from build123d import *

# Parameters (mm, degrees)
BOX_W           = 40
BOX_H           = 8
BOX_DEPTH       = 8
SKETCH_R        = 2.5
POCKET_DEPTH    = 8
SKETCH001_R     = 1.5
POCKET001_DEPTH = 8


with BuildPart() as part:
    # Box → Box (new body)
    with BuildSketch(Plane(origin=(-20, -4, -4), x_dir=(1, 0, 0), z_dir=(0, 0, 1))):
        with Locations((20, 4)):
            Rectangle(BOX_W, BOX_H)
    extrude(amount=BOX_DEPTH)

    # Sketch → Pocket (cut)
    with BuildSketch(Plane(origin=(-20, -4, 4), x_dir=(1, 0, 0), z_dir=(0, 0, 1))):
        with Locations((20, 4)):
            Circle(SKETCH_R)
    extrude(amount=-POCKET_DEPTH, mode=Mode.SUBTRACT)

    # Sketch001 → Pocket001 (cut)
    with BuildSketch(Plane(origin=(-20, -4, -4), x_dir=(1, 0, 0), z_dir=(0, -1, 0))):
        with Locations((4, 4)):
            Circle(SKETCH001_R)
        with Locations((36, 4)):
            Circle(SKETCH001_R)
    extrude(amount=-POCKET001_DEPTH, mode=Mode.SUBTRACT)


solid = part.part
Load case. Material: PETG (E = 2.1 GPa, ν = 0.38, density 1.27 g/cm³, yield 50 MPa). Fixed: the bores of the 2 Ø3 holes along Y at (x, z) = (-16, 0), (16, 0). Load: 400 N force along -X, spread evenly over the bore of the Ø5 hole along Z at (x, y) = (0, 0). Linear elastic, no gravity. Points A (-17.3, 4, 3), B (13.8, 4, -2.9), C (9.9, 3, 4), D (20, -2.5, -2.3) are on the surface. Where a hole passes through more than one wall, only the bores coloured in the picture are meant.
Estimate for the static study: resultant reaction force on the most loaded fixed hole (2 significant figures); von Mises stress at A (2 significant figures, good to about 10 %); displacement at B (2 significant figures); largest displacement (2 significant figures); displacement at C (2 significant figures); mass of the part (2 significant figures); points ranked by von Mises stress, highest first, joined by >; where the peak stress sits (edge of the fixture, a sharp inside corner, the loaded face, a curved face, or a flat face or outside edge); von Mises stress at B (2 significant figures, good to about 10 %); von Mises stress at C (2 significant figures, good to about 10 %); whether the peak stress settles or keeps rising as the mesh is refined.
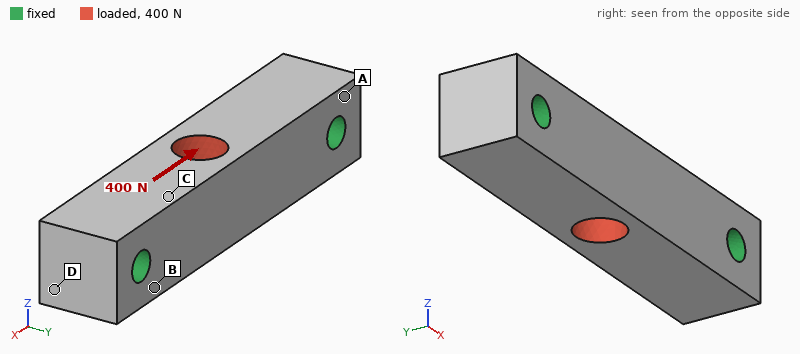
200 N
1.2 MPa
5.3 µm
24 µm
9.7 µm
2.9 g
C > B > A > D
edge of the fixture
2.0 MPa
2.8 MPa
keeps rising
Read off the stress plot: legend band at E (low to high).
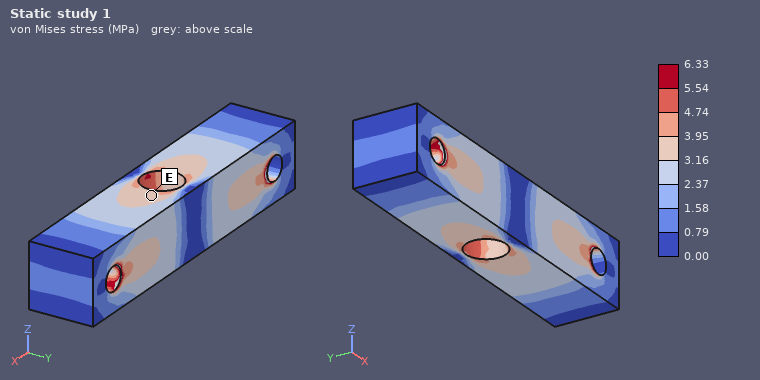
3.16 to 3.95 MPa
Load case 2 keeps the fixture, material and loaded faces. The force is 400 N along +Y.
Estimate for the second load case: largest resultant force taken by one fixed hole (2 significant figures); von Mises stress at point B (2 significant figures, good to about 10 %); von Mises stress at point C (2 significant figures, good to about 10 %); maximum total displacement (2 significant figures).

200 N
9.8 MPa
5.3 MPa
0.16 mm
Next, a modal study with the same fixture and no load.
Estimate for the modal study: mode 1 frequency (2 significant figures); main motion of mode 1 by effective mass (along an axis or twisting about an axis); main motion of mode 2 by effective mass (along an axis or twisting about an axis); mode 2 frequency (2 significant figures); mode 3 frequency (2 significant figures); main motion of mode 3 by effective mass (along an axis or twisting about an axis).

6700 Hz
along Z
along Y
8600 Hz
12 kHz
twisting about X
